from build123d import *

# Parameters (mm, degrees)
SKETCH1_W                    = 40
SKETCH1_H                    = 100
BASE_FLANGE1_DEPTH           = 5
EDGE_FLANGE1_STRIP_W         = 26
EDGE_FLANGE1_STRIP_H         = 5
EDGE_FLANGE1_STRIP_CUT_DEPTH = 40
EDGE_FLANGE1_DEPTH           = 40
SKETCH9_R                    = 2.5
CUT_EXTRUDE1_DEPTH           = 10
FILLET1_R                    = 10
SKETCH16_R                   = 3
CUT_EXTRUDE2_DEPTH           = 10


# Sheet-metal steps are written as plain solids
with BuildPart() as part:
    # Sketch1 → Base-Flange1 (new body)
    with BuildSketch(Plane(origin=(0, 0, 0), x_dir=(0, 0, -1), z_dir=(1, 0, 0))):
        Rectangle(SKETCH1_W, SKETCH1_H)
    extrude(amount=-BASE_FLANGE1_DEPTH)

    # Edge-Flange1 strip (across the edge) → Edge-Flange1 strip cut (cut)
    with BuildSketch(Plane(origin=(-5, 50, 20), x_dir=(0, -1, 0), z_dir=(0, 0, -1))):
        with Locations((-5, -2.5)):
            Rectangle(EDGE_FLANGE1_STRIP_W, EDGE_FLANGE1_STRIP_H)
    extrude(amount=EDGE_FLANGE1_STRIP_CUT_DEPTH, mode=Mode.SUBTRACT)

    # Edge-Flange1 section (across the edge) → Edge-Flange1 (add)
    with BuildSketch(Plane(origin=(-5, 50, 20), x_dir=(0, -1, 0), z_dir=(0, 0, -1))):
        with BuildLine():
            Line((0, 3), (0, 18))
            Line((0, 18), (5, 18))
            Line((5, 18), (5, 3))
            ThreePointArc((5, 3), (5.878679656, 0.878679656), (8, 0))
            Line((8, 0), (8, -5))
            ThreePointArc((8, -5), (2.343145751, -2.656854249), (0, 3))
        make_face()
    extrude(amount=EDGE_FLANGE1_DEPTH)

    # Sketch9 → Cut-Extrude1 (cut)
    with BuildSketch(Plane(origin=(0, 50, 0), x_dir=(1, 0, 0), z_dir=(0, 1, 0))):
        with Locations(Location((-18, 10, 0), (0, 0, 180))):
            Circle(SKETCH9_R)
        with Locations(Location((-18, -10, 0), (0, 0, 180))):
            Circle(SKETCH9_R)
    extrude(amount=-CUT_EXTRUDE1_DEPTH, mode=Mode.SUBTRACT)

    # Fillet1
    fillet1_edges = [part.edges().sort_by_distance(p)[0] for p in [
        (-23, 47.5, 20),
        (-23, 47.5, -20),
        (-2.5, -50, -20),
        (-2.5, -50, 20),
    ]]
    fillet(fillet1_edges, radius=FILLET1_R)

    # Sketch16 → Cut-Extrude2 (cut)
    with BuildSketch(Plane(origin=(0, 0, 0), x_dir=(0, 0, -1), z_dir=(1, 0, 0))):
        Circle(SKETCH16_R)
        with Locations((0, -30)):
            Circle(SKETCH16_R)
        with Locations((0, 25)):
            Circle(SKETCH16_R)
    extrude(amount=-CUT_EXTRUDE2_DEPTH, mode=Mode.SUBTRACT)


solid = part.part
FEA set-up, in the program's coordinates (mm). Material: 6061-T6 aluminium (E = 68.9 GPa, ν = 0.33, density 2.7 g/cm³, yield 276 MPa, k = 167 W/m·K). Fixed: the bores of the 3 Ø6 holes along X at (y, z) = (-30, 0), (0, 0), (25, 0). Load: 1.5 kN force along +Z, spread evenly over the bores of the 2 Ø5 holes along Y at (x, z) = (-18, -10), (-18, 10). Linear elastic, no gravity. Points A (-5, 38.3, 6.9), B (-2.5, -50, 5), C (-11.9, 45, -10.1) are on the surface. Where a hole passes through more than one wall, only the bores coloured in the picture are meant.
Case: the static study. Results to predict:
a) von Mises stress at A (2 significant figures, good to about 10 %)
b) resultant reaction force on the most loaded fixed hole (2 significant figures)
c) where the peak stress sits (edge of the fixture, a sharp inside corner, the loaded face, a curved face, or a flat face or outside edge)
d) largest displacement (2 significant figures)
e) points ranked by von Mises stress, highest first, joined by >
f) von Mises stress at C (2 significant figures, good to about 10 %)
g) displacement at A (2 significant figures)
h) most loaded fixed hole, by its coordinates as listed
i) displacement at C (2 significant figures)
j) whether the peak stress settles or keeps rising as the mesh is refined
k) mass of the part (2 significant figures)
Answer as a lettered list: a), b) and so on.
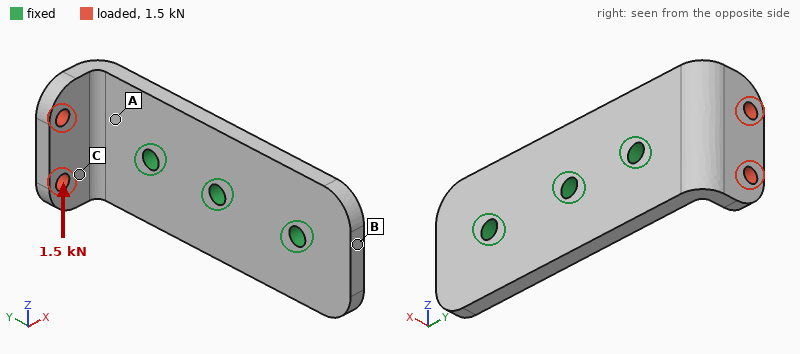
a) 99 MPa
b) 2.2 kN
c) edge of the fixture
d) 0.28 mm
e) A > C > B
f) 55 MPa
g) 0.058 mm
h) (25, 0)
i) 0.16 mm
j) keeps rising
k) 60 g
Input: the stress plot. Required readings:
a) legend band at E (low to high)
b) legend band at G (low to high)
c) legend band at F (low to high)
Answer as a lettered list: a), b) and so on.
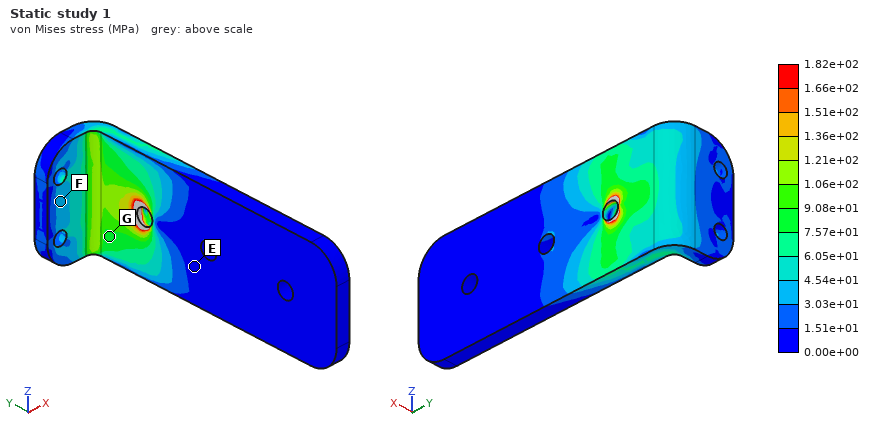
a) 0.00e+00 to 1.51e+01 MPa
b) 7.57e+01 to 9.08e+01 MPa
c) 3.03e+01 to 4.54e+01 MPa
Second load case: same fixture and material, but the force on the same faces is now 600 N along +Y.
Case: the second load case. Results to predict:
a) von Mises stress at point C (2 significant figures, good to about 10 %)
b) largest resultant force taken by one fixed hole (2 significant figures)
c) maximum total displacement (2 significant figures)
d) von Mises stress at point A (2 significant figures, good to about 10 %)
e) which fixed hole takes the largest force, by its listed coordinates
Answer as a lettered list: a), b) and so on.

a) 21 MPa
b) 480 N
c) 0.20 mm
d) 55 MPa
e) (25, 0)
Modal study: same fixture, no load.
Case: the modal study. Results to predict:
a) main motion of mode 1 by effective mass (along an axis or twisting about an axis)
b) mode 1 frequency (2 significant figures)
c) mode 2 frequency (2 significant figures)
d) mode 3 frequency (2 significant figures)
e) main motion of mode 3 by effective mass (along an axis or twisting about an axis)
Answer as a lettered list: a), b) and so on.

a) along X
b) 3200 Hz
c) 4200 Hz
d) 8700 Hz
e) twisting about Y
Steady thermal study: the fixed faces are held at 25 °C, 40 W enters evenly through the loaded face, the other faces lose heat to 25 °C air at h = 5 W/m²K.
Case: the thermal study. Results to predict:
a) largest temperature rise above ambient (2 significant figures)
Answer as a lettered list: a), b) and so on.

a) 52 K
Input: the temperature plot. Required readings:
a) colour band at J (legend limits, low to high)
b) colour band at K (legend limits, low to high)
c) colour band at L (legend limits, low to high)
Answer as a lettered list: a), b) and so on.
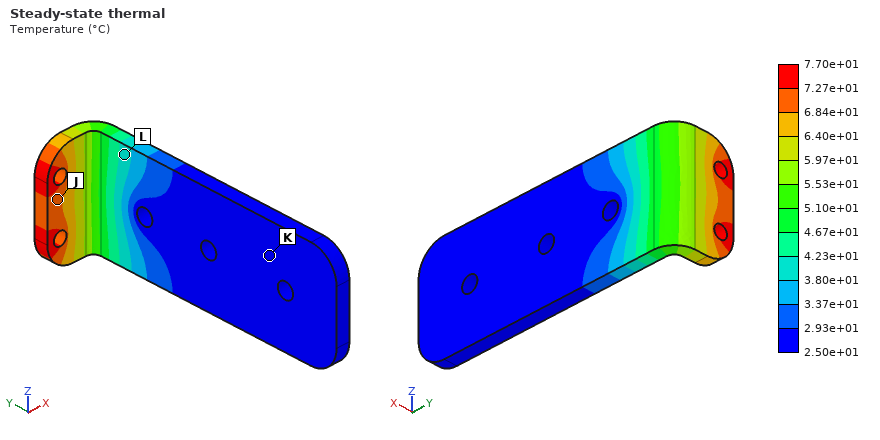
a) 6.84e+01 to 7.27e+01 °C
b) 2.50e+01 to 2.93e+01 °C
c) 3.80e+01 to 4.23e+01 °C
